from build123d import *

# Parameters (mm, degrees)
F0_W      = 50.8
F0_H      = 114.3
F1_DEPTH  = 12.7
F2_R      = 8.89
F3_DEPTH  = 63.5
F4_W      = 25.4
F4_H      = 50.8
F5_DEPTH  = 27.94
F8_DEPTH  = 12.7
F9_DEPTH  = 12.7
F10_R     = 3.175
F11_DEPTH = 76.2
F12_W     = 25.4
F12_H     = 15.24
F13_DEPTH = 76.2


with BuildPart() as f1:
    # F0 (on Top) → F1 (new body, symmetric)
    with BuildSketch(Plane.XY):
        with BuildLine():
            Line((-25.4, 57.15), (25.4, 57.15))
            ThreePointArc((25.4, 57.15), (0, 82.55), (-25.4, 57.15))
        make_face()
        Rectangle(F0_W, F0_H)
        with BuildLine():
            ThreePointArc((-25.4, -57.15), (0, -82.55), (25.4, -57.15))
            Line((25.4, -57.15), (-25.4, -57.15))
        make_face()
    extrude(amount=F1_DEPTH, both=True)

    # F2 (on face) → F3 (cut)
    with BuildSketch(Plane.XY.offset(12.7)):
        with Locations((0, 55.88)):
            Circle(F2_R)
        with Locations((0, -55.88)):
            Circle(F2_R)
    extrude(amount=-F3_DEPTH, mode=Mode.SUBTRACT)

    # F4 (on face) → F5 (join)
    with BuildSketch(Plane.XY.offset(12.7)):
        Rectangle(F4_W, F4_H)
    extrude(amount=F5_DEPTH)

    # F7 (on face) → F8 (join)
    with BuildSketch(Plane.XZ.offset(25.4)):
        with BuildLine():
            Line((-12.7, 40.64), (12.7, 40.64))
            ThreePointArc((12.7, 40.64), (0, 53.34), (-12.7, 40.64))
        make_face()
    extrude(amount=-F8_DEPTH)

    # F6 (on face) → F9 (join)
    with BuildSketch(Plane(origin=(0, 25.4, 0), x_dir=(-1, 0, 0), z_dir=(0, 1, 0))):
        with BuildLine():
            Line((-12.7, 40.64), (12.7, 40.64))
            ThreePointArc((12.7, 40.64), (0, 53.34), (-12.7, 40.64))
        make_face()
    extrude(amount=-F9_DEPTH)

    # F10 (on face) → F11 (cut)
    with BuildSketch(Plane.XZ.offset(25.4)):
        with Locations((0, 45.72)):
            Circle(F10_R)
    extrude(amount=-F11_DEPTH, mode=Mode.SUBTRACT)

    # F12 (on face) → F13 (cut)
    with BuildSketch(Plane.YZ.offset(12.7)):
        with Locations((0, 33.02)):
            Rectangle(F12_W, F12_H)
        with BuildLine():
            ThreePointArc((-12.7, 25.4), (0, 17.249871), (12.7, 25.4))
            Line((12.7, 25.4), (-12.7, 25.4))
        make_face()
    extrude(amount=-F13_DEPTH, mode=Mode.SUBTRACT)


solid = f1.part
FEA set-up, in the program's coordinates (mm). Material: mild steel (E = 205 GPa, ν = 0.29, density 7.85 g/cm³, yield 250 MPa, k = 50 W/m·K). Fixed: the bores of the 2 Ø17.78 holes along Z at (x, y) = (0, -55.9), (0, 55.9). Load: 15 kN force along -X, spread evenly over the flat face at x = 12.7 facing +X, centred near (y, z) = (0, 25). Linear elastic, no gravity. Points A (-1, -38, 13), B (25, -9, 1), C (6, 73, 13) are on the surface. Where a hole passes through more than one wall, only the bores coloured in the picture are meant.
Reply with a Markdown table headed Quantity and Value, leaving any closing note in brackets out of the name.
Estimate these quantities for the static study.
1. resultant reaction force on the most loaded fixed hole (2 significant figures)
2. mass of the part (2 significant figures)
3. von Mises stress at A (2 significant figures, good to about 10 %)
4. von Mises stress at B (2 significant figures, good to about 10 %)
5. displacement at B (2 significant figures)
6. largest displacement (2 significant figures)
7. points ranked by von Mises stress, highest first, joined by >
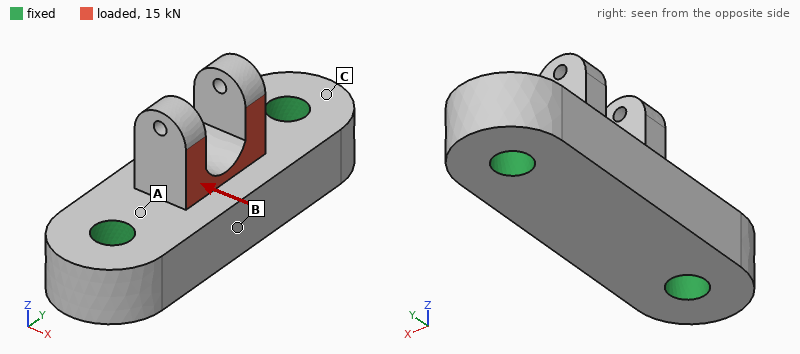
| Quantity | Value |
|---|---|
| resultant reaction force on the most loaded fixed hole | 7.5 kN |
| mass of the part | 1.7 kg |
| von Mises stress at A | 46 MPa |
| von Mises stress at B | 17 MPa |
| displacement at B | 11 µm |
| largest displacement | 38 µm |
| points ranked by von Mises stress, highest first, joined by > | A > B > C |
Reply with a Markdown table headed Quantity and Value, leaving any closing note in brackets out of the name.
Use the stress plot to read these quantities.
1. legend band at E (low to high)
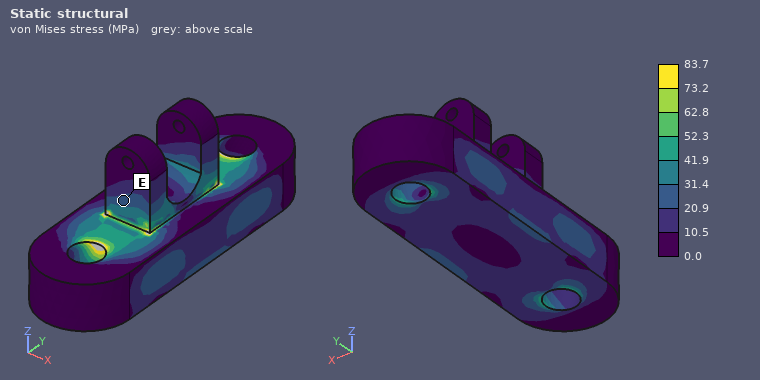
| Quantity | Value |
|---|---|
| legend band at E | 20.9 to 31.4 MPa |
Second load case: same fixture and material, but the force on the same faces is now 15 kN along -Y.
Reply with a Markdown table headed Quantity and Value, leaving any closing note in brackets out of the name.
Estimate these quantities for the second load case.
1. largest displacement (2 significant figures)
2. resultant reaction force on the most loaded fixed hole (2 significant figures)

| Quantity | Value |
|---|---|
| largest displacement | 31 µm |
| resultant reaction force on the most loaded fixed hole | 8.8 kN |
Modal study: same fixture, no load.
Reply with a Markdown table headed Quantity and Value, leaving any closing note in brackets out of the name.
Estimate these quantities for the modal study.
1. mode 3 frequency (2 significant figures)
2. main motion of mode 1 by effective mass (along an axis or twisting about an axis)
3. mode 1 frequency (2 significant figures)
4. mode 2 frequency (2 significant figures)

| Quantity | Value |
|---|---|
| mode 3 frequency | 7900 Hz |
| main motion of mode 1 by effective mass | along X |
| mode 1 frequency | 6500 Hz |
| mode 2 frequency | 7600 Hz |
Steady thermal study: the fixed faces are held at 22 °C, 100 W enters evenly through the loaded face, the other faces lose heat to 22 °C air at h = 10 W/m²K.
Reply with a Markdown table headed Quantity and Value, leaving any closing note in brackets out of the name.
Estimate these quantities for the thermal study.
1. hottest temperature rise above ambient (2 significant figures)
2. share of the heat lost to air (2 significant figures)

| Quantity | Value |
|---|---|
| hottest temperature rise above ambient | 78 K |
| share of the heat lost to air | 6.0 % |
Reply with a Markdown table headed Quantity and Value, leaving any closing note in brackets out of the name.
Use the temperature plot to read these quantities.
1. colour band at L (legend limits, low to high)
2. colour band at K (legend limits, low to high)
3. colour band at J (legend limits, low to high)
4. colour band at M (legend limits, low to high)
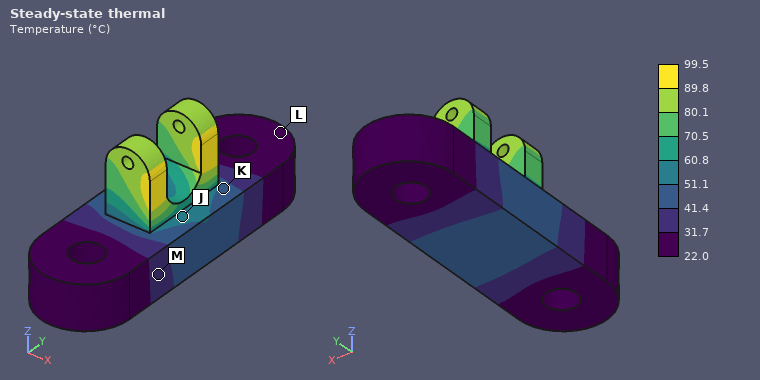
| Quantity | Value |
|---|---|
| colour band at L | 22.0 to 31.7 °C |
| colour band at K | 41.4 to 51.1 °C |
| colour band at J | 51.1 to 60.8 °C |
| colour band at M | 31.7 to 41.4 °C |
